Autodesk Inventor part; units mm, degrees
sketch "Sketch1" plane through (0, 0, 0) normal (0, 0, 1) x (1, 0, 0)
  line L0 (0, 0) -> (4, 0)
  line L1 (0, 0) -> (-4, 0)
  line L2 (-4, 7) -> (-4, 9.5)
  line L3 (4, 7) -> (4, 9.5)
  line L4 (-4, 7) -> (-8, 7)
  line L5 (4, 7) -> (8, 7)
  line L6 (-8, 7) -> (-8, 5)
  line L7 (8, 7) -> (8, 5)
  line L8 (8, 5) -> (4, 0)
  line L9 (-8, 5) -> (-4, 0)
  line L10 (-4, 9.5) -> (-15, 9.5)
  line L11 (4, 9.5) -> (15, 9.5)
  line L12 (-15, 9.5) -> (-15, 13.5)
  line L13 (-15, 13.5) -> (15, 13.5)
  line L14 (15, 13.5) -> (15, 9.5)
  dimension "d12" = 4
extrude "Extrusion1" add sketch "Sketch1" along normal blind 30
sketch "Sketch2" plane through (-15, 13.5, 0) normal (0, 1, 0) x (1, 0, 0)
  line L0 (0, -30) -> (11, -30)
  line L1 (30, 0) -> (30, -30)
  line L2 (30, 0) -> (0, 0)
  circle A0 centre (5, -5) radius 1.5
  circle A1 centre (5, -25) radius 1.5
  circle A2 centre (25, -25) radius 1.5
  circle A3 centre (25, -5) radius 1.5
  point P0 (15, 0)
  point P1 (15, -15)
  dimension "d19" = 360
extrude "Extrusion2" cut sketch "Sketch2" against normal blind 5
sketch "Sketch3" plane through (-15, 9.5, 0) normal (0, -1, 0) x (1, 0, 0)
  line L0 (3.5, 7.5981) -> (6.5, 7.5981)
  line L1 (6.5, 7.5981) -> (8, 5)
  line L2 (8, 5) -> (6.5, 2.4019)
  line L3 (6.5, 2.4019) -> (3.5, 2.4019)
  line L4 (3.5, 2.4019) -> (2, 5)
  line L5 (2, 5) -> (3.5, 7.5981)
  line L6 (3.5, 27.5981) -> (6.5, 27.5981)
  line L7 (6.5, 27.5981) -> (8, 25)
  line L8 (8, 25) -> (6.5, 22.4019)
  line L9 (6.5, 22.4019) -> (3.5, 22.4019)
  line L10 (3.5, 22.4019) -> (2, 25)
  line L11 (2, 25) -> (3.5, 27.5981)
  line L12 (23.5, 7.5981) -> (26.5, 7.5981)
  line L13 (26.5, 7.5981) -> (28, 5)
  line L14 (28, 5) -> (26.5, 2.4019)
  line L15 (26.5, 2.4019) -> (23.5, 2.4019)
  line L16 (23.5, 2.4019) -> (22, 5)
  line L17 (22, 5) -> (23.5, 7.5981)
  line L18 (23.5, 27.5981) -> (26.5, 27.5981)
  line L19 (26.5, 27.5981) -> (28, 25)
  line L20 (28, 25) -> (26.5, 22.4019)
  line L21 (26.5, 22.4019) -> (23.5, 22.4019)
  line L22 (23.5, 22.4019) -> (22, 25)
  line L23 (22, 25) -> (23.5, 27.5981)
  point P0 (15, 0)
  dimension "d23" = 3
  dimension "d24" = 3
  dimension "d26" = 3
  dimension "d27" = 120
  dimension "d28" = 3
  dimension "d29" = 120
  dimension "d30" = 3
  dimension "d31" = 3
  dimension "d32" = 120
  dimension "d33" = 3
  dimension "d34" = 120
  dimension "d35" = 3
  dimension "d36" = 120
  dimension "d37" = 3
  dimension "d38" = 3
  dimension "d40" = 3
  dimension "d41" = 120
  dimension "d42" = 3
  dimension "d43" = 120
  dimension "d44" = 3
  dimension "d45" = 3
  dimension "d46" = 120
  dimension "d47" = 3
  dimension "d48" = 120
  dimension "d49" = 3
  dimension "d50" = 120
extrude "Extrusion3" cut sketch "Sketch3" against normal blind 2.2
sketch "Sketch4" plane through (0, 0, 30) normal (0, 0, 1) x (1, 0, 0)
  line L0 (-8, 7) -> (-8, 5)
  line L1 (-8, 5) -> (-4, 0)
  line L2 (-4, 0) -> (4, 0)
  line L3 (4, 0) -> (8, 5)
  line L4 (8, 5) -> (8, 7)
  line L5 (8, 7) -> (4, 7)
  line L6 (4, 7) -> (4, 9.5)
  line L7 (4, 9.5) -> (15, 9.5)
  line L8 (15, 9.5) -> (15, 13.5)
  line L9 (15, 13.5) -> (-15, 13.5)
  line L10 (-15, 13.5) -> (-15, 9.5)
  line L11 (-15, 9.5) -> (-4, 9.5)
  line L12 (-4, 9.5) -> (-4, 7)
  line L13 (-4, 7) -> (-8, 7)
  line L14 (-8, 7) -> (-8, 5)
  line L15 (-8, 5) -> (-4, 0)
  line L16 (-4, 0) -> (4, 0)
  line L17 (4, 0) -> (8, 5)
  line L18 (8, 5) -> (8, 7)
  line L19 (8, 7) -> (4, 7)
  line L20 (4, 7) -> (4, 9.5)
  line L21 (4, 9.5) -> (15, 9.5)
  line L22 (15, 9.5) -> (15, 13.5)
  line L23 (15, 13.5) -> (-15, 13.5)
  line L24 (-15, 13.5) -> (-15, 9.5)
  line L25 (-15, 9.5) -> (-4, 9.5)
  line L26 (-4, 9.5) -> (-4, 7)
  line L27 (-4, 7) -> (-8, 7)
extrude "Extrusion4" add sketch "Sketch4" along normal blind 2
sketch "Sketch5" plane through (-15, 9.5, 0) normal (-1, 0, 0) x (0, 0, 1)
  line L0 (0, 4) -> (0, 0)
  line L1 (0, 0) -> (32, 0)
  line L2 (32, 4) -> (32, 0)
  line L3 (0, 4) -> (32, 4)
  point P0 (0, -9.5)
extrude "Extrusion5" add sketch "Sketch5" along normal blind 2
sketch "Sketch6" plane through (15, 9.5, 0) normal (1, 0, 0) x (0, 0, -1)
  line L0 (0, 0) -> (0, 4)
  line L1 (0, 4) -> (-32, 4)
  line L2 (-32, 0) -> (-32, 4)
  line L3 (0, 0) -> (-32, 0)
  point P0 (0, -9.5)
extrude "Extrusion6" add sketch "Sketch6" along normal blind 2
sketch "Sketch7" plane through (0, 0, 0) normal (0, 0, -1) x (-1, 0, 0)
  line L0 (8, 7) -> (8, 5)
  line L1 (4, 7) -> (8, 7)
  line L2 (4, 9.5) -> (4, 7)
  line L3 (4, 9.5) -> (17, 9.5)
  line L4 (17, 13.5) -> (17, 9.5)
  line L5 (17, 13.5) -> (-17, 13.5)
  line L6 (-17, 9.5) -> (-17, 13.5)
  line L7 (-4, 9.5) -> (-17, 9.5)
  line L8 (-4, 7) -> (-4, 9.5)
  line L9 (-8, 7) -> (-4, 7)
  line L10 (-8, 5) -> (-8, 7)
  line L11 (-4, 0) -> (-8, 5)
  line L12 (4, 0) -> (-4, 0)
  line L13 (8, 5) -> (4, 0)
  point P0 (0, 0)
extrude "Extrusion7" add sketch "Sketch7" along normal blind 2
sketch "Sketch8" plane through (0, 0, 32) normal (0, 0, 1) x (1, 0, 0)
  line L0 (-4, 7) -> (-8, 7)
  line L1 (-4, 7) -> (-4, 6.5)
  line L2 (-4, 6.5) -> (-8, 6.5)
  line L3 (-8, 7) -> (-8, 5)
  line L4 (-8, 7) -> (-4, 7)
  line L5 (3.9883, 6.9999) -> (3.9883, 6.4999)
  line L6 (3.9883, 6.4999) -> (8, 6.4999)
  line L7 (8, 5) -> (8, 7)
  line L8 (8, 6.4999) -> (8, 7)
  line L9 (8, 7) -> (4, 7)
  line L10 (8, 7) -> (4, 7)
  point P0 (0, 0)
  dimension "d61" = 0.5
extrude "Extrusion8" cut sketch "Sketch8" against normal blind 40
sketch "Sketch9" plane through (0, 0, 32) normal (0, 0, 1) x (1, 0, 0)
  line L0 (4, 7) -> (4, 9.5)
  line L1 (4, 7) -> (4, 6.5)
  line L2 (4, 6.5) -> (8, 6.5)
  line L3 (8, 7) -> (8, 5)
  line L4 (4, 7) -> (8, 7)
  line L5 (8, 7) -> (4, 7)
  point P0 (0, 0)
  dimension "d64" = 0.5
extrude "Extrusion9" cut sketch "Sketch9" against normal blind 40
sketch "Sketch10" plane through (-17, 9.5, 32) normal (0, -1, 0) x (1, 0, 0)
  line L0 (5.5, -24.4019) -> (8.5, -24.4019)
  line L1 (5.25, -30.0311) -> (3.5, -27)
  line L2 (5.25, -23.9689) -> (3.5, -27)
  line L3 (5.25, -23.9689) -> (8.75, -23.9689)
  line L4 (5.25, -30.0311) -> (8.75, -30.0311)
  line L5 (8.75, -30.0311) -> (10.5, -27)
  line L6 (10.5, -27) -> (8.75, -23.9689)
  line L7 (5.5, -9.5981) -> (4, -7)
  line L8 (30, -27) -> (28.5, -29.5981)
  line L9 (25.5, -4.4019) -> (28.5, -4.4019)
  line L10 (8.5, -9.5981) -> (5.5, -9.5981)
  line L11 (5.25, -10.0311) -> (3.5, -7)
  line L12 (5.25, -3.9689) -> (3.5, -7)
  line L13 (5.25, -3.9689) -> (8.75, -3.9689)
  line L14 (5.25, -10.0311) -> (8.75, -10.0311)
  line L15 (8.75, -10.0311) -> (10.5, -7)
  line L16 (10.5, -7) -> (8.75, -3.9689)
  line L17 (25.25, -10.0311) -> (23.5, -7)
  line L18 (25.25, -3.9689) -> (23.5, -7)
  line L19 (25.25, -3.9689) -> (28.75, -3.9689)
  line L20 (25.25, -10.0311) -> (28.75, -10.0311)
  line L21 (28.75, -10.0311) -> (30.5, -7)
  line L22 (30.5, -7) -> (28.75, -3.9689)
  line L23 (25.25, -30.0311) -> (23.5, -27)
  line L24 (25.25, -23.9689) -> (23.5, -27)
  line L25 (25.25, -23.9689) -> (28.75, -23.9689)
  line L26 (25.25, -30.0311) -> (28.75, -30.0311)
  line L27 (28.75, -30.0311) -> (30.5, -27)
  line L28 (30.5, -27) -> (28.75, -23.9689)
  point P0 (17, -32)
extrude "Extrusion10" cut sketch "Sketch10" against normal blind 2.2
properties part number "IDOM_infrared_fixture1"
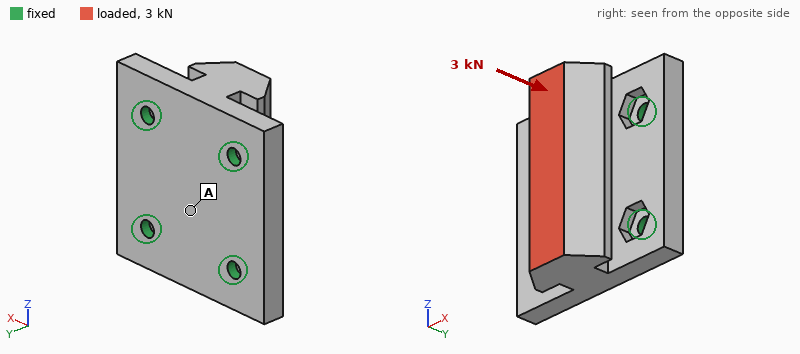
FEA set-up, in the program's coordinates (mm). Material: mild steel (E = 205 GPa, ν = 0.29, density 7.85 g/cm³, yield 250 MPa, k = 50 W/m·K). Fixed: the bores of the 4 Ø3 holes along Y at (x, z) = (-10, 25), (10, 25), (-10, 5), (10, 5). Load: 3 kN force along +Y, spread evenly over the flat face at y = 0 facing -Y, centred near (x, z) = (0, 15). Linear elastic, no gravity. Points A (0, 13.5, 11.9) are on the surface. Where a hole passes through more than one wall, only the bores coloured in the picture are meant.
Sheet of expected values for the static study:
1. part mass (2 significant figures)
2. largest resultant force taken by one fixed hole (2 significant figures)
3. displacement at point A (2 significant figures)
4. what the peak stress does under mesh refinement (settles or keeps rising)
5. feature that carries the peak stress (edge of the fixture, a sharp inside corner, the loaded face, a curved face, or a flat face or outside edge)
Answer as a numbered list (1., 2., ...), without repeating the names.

1. 63 g
2. 940 N
3. 5.7 µm
4. keeps rising
5. edge of the fixture
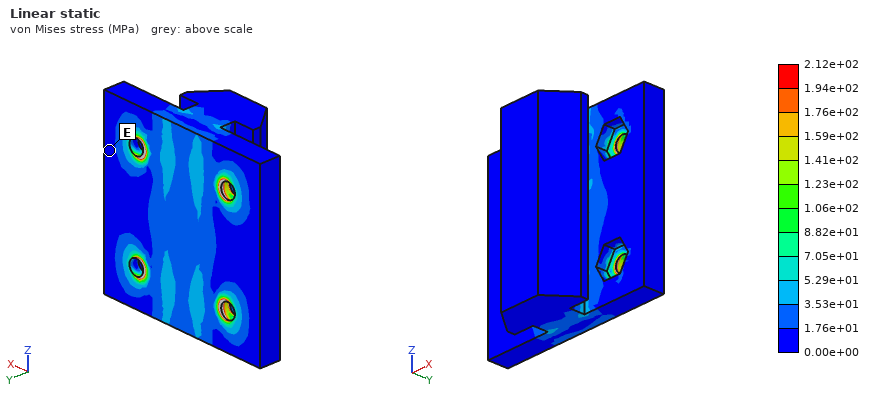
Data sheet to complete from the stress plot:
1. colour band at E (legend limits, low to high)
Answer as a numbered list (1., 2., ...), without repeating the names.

1. 0.00e+00 to 1.76e+01 MPa
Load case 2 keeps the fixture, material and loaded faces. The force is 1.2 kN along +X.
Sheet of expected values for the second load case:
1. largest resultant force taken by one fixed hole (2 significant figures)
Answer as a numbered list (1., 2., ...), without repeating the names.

1. 520 N
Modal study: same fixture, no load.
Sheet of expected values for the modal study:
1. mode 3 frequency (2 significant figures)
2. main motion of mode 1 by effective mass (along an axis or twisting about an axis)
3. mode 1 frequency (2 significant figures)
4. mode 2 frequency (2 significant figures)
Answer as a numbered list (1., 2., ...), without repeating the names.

1. 18 kHz
2. along Z
3. 15 kHz
4. 18 kHz
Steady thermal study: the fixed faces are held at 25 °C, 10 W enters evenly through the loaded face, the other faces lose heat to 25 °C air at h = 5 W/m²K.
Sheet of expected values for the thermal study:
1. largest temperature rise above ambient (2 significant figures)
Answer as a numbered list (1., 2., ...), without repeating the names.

1. 16 K
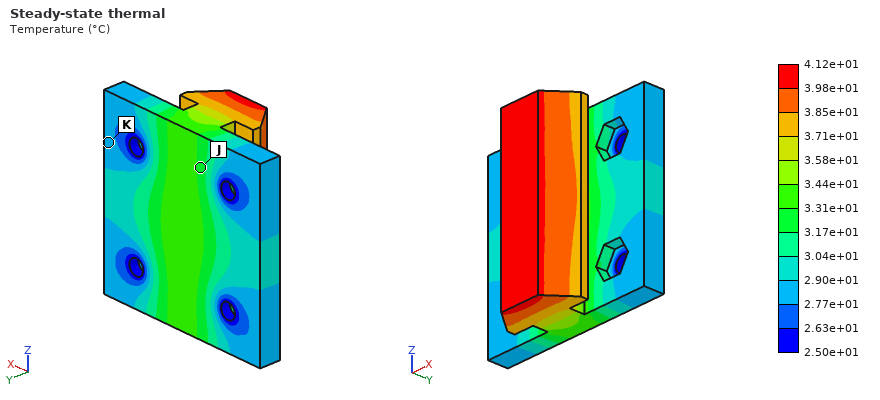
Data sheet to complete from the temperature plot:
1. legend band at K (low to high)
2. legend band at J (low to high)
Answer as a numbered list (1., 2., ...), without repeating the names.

1. 2.77e+01 to 2.90e+01 °C
2. 3.17e+01 to 3.31e+01 °C
